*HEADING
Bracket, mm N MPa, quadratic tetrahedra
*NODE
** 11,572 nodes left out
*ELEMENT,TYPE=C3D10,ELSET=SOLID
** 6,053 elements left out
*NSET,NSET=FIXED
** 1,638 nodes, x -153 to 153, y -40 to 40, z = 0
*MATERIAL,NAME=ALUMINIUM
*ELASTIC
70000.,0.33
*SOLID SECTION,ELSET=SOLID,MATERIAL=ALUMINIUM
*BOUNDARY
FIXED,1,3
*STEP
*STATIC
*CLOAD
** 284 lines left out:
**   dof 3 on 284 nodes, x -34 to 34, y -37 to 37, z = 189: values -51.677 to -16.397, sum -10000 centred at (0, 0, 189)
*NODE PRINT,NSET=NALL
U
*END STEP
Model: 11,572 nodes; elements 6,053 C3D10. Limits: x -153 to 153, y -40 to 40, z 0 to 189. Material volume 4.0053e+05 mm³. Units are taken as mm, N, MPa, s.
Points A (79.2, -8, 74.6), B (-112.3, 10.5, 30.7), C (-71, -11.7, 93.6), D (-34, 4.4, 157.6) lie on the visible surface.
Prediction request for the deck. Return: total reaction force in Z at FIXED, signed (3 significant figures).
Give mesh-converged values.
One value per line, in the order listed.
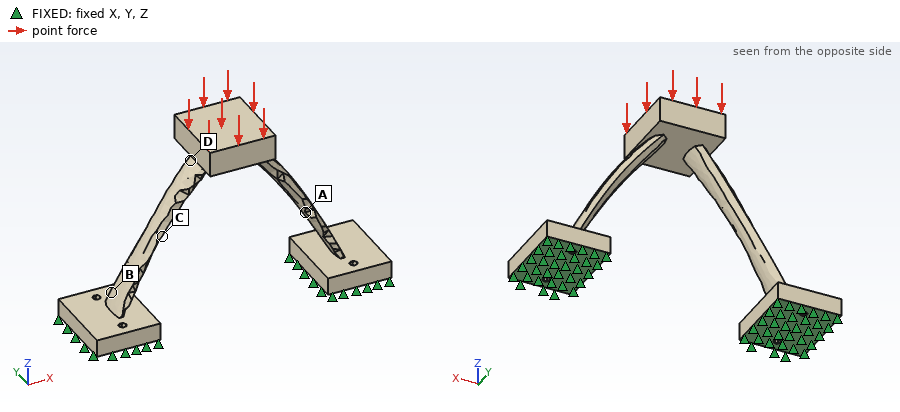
10000 N
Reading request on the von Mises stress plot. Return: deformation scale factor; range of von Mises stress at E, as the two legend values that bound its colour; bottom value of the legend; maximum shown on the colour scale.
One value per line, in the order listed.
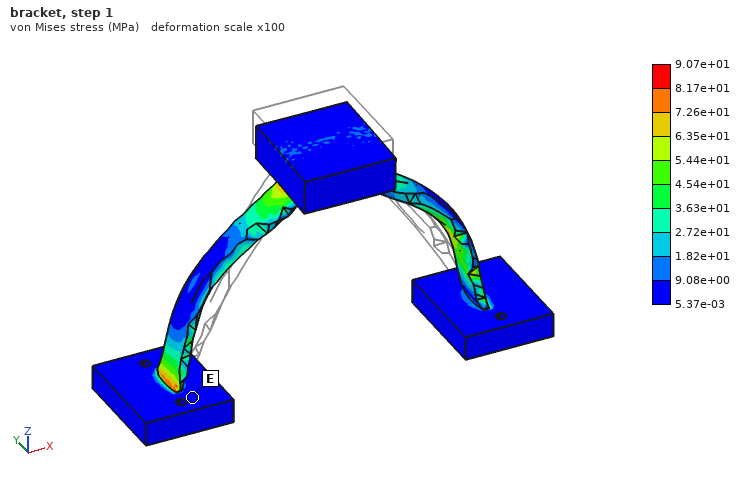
100
5.37e-03 to 9.08e+00 MPa
5.37e-03 MPa
9.07e+01 MPa
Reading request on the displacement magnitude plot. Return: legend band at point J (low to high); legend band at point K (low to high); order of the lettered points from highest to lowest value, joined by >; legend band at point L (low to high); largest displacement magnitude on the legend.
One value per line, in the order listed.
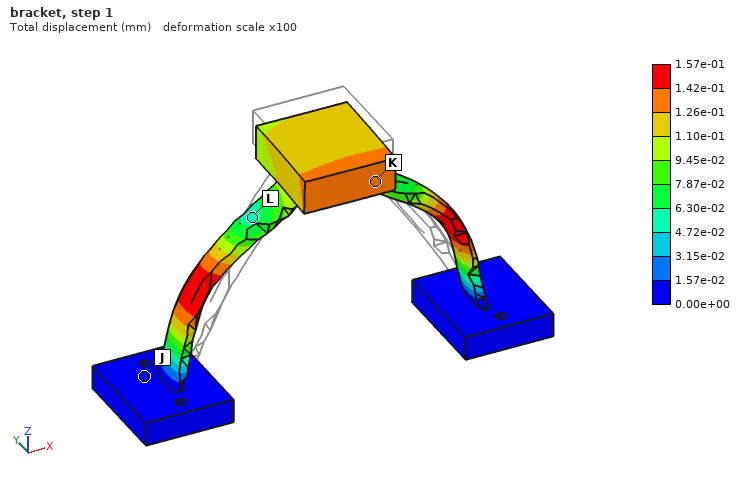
0.00e+00 to 1.57e-02 mm
1.26e-01 to 1.42e-01 mm
K > L > J
4.72e-02 to 6.30e-02 mm
1.57e-01 mm
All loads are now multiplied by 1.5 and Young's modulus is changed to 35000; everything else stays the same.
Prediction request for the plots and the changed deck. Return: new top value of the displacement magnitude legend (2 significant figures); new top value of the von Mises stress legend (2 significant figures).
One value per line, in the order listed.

0.47 mm
140 MPa
